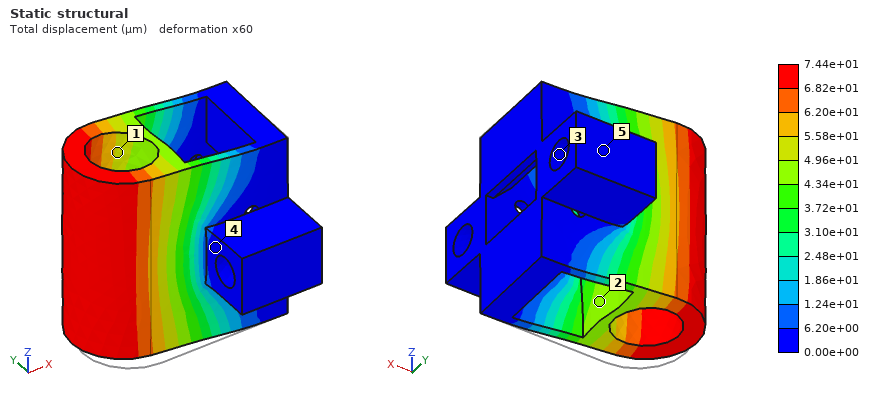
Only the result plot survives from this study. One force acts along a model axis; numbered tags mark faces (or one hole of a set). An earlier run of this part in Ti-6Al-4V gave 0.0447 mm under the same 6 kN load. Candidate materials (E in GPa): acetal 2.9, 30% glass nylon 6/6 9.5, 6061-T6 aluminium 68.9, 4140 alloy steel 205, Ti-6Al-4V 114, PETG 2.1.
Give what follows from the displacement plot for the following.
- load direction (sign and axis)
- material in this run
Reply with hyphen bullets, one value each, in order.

- +Y
- 6061-T6 aluminium
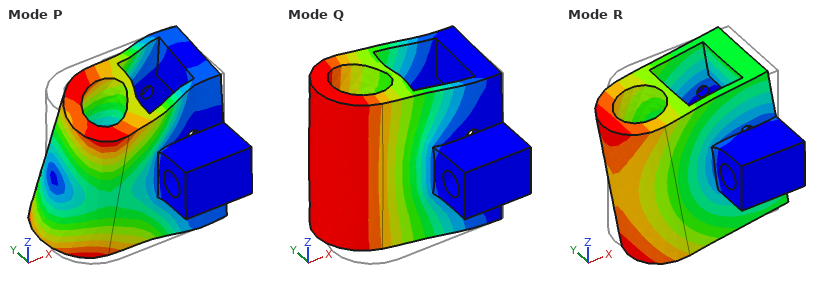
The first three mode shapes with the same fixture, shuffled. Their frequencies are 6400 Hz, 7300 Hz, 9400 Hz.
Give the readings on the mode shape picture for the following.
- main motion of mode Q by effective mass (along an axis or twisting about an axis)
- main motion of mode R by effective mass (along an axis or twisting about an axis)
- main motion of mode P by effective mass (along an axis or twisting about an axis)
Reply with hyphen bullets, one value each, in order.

- along Y
- along Z
- twisting about X
